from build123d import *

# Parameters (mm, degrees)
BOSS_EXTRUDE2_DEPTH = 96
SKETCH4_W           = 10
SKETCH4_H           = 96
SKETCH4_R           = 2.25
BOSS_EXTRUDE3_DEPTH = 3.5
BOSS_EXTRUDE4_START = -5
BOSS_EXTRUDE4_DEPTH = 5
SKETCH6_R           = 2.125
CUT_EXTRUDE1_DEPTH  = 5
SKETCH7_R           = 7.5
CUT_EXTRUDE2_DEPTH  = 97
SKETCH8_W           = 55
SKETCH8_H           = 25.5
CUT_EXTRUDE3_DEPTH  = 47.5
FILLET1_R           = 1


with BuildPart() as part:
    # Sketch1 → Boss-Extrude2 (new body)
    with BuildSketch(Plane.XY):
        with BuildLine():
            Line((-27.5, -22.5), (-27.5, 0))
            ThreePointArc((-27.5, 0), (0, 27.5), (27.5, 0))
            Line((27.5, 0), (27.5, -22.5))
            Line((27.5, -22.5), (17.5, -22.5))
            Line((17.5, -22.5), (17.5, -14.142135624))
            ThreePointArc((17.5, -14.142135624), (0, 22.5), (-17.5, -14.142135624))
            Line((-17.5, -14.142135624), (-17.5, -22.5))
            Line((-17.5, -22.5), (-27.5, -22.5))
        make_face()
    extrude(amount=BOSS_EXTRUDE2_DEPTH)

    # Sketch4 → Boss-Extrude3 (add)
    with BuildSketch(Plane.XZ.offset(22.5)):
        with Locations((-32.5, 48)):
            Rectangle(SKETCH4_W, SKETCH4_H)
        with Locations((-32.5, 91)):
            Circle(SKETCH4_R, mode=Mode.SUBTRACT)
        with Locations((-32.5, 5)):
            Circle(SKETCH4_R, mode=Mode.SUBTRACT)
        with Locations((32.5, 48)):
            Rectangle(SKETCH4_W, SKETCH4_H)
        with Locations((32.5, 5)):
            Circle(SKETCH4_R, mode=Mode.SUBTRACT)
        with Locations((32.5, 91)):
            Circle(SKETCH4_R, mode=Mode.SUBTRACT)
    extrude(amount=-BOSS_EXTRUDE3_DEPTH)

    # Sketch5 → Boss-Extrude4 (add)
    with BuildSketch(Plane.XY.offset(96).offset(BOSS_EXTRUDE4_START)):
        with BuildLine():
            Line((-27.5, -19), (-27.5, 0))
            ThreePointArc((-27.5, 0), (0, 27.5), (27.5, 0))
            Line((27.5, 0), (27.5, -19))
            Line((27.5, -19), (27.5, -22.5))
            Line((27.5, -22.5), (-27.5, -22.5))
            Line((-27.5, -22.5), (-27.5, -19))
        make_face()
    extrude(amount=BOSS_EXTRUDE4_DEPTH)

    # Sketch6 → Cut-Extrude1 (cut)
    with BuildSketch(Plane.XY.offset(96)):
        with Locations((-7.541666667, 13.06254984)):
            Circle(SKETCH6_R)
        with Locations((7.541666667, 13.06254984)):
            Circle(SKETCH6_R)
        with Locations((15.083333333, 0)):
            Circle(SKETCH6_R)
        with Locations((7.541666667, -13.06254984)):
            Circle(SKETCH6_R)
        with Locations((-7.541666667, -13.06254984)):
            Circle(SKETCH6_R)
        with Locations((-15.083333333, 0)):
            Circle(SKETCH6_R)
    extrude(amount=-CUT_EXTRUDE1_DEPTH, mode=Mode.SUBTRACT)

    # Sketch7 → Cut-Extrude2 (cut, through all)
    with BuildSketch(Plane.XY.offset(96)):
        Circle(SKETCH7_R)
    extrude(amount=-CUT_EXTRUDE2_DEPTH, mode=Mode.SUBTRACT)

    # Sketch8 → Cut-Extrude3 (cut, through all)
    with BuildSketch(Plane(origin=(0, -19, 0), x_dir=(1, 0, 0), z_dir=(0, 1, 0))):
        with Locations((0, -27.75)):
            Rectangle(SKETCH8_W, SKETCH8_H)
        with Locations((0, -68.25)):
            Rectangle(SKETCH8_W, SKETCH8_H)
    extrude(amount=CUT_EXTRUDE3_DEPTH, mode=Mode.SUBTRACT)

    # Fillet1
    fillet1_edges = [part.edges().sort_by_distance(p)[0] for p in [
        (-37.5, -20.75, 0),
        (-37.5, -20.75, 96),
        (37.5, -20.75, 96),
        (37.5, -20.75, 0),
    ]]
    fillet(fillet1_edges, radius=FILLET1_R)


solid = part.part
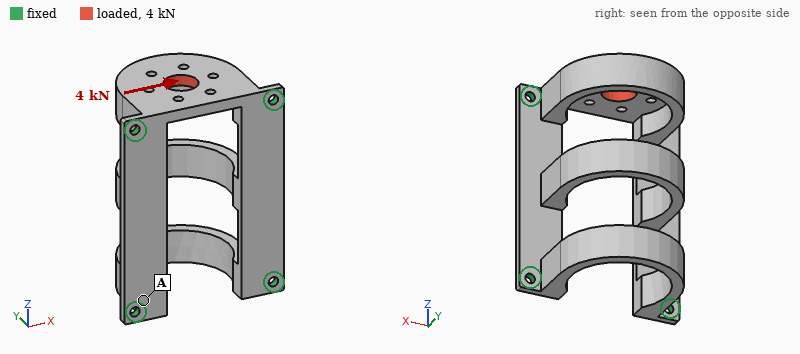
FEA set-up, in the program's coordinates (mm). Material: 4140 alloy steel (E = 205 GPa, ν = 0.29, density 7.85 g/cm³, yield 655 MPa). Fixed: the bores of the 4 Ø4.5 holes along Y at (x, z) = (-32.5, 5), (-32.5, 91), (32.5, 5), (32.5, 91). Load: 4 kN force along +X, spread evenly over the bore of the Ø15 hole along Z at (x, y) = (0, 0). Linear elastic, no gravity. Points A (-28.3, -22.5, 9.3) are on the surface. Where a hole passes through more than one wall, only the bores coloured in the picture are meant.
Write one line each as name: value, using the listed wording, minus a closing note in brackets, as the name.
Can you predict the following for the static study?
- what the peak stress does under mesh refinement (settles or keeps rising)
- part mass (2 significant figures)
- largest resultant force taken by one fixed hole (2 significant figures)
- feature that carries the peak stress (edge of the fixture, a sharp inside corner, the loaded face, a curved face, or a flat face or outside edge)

what the peak stress does under mesh refinement: keeps rising
part mass: 400 g
largest resultant force taken by one fixed hole: 2.5 kN
feature that carries the peak stress: edge of the fixture
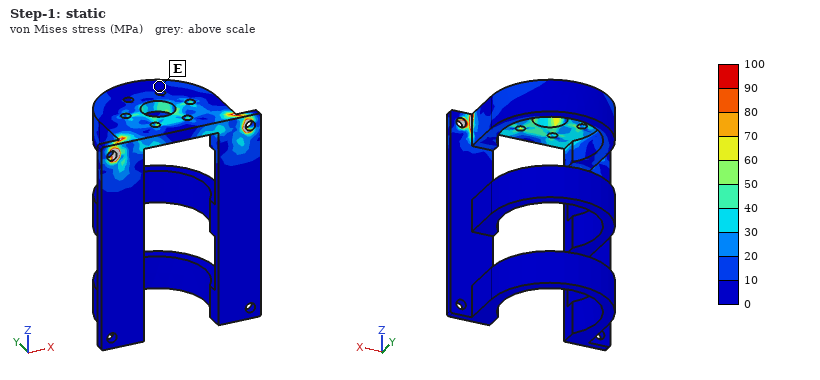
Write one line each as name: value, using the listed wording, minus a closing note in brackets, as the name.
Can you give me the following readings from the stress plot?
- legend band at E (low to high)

legend band at E: 0 to 10 MPa
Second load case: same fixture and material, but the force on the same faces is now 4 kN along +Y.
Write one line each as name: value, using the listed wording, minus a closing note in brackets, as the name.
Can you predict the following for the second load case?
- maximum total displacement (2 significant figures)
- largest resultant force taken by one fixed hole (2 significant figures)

maximum total displacement: 77 µm
largest resultant force taken by one fixed hole: 2.3 kN
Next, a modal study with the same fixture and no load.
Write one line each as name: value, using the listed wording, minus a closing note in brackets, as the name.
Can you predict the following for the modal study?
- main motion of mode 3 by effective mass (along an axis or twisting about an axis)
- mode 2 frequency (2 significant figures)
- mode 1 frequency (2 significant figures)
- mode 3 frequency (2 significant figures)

main motion of mode 3 by effective mass: along X
mode 2 frequency: 1400 Hz
mode 1 frequency: 1300 Hz
mode 3 frequency: 1500 Hz
